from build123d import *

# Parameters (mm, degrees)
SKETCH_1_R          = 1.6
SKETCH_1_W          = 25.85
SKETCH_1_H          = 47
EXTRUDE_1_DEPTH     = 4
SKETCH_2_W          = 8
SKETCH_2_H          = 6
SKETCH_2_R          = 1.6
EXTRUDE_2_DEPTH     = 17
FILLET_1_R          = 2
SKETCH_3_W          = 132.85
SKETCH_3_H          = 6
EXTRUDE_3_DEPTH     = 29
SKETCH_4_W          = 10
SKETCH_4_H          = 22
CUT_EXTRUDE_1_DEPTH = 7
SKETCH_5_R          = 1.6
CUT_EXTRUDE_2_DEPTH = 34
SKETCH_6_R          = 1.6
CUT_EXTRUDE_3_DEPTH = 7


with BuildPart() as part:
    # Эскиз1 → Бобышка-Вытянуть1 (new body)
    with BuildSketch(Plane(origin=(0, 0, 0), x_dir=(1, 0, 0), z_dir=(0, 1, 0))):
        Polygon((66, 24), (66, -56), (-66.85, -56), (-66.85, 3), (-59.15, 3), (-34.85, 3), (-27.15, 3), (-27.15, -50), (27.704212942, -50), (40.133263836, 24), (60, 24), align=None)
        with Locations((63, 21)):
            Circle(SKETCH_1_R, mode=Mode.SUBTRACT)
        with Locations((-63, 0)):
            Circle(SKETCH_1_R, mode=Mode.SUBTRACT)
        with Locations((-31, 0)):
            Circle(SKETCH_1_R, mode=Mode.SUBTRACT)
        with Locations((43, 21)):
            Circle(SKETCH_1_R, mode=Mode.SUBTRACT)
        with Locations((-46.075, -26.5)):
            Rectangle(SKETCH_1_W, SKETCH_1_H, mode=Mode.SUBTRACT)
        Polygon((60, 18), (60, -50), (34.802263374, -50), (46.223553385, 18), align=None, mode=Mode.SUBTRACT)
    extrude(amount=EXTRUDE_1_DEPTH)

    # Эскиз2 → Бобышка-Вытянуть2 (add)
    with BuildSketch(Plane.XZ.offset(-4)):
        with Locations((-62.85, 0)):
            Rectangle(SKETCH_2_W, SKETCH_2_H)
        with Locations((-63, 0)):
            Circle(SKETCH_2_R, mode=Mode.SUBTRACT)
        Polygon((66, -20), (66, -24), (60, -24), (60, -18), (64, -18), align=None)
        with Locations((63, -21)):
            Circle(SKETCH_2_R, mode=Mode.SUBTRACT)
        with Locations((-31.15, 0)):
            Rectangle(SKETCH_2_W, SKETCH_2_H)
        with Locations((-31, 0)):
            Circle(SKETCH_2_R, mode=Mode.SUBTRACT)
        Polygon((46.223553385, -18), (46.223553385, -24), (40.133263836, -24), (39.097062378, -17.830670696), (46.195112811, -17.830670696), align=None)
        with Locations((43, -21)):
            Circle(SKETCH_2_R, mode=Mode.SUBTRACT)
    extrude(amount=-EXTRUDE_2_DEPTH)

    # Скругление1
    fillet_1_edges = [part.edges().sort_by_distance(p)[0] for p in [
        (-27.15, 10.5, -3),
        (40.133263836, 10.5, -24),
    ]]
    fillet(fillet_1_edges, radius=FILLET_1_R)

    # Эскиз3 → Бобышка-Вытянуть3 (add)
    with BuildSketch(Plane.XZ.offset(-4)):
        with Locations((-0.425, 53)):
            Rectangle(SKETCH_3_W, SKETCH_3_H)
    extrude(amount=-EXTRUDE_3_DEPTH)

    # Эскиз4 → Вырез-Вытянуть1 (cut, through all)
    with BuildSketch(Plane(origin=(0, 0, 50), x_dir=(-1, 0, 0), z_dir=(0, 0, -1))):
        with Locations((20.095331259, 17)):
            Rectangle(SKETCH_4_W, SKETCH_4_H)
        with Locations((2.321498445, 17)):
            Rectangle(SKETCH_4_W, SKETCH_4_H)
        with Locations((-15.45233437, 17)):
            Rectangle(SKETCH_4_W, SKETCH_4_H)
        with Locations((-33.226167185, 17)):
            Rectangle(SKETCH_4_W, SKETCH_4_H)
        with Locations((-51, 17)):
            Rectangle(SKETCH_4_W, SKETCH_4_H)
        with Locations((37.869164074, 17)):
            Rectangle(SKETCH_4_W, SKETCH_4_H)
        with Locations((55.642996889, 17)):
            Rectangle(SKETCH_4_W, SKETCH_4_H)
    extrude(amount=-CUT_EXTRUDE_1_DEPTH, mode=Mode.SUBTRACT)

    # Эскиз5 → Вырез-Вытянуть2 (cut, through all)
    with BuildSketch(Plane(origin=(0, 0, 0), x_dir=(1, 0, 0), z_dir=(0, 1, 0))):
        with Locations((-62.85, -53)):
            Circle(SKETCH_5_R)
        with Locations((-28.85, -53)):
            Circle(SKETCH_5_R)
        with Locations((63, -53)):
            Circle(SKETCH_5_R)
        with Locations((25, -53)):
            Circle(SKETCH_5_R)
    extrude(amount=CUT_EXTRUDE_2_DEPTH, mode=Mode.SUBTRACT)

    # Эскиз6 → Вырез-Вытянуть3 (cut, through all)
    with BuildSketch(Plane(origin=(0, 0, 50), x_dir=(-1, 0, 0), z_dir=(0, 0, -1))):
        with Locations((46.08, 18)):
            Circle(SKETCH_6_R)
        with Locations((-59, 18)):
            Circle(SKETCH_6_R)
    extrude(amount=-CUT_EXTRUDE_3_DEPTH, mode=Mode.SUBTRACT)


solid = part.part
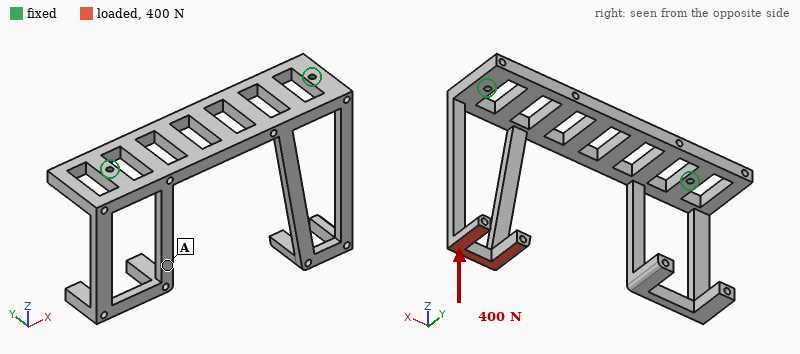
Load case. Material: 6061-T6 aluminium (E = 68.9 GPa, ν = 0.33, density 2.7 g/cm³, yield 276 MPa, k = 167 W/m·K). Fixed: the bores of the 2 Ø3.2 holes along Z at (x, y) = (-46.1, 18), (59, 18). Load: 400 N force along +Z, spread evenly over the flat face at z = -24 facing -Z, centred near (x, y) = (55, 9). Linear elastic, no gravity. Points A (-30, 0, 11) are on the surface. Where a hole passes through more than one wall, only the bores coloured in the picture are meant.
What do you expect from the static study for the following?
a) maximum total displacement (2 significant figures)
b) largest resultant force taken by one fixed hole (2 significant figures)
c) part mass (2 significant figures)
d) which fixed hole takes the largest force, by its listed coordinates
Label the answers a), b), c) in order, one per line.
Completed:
a) 1.8 mm
b) 380 N
c) 70 g
d) (59, 18)
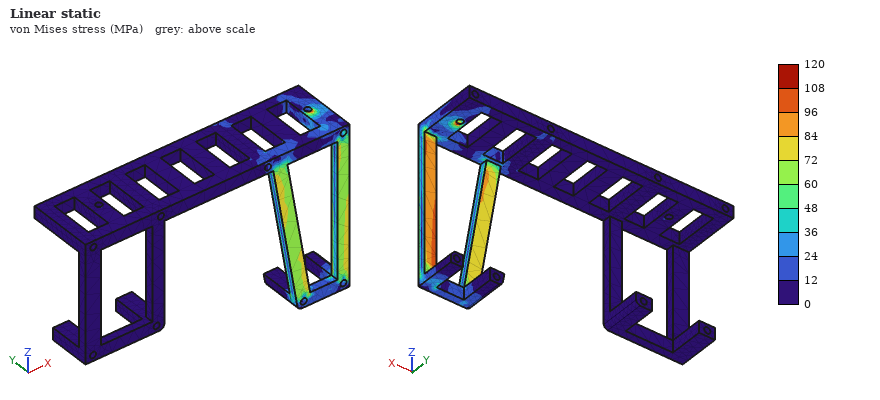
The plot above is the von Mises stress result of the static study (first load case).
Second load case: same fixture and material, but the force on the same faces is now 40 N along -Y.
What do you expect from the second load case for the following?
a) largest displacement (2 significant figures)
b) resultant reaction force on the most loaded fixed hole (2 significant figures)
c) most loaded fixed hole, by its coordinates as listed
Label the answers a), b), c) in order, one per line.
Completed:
a) 1.5 mm
b) 38 N
c) (59, 18)
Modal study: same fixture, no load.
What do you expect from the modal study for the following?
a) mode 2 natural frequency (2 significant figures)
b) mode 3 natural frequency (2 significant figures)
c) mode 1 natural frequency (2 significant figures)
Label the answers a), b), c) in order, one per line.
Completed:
a) 530 Hz
b) 730 Hz
c) 350 Hz
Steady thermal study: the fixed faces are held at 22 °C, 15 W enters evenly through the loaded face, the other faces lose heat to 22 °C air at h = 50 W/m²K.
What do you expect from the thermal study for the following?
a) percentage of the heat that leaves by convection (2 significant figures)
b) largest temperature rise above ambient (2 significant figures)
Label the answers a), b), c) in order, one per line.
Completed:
a) 73 %
b) 77 K
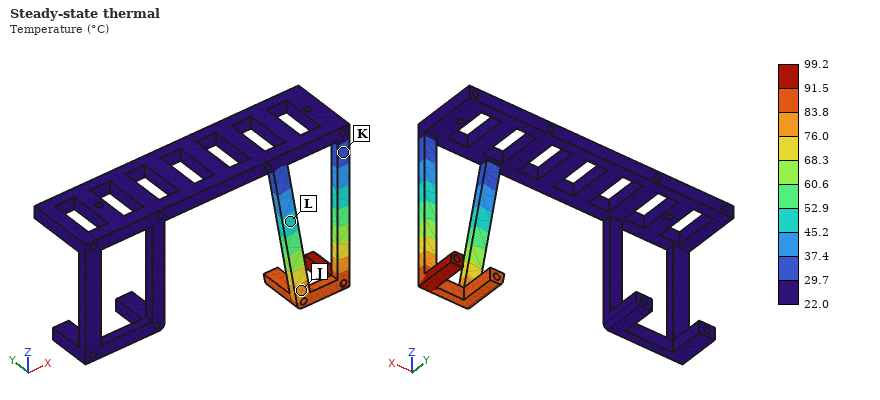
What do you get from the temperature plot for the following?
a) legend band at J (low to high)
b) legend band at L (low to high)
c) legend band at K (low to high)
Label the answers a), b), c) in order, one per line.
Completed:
a) 76.0 to 83.8 °C
b) 45.2 to 52.9 °C
c) 29.7 to 37.4 °C
